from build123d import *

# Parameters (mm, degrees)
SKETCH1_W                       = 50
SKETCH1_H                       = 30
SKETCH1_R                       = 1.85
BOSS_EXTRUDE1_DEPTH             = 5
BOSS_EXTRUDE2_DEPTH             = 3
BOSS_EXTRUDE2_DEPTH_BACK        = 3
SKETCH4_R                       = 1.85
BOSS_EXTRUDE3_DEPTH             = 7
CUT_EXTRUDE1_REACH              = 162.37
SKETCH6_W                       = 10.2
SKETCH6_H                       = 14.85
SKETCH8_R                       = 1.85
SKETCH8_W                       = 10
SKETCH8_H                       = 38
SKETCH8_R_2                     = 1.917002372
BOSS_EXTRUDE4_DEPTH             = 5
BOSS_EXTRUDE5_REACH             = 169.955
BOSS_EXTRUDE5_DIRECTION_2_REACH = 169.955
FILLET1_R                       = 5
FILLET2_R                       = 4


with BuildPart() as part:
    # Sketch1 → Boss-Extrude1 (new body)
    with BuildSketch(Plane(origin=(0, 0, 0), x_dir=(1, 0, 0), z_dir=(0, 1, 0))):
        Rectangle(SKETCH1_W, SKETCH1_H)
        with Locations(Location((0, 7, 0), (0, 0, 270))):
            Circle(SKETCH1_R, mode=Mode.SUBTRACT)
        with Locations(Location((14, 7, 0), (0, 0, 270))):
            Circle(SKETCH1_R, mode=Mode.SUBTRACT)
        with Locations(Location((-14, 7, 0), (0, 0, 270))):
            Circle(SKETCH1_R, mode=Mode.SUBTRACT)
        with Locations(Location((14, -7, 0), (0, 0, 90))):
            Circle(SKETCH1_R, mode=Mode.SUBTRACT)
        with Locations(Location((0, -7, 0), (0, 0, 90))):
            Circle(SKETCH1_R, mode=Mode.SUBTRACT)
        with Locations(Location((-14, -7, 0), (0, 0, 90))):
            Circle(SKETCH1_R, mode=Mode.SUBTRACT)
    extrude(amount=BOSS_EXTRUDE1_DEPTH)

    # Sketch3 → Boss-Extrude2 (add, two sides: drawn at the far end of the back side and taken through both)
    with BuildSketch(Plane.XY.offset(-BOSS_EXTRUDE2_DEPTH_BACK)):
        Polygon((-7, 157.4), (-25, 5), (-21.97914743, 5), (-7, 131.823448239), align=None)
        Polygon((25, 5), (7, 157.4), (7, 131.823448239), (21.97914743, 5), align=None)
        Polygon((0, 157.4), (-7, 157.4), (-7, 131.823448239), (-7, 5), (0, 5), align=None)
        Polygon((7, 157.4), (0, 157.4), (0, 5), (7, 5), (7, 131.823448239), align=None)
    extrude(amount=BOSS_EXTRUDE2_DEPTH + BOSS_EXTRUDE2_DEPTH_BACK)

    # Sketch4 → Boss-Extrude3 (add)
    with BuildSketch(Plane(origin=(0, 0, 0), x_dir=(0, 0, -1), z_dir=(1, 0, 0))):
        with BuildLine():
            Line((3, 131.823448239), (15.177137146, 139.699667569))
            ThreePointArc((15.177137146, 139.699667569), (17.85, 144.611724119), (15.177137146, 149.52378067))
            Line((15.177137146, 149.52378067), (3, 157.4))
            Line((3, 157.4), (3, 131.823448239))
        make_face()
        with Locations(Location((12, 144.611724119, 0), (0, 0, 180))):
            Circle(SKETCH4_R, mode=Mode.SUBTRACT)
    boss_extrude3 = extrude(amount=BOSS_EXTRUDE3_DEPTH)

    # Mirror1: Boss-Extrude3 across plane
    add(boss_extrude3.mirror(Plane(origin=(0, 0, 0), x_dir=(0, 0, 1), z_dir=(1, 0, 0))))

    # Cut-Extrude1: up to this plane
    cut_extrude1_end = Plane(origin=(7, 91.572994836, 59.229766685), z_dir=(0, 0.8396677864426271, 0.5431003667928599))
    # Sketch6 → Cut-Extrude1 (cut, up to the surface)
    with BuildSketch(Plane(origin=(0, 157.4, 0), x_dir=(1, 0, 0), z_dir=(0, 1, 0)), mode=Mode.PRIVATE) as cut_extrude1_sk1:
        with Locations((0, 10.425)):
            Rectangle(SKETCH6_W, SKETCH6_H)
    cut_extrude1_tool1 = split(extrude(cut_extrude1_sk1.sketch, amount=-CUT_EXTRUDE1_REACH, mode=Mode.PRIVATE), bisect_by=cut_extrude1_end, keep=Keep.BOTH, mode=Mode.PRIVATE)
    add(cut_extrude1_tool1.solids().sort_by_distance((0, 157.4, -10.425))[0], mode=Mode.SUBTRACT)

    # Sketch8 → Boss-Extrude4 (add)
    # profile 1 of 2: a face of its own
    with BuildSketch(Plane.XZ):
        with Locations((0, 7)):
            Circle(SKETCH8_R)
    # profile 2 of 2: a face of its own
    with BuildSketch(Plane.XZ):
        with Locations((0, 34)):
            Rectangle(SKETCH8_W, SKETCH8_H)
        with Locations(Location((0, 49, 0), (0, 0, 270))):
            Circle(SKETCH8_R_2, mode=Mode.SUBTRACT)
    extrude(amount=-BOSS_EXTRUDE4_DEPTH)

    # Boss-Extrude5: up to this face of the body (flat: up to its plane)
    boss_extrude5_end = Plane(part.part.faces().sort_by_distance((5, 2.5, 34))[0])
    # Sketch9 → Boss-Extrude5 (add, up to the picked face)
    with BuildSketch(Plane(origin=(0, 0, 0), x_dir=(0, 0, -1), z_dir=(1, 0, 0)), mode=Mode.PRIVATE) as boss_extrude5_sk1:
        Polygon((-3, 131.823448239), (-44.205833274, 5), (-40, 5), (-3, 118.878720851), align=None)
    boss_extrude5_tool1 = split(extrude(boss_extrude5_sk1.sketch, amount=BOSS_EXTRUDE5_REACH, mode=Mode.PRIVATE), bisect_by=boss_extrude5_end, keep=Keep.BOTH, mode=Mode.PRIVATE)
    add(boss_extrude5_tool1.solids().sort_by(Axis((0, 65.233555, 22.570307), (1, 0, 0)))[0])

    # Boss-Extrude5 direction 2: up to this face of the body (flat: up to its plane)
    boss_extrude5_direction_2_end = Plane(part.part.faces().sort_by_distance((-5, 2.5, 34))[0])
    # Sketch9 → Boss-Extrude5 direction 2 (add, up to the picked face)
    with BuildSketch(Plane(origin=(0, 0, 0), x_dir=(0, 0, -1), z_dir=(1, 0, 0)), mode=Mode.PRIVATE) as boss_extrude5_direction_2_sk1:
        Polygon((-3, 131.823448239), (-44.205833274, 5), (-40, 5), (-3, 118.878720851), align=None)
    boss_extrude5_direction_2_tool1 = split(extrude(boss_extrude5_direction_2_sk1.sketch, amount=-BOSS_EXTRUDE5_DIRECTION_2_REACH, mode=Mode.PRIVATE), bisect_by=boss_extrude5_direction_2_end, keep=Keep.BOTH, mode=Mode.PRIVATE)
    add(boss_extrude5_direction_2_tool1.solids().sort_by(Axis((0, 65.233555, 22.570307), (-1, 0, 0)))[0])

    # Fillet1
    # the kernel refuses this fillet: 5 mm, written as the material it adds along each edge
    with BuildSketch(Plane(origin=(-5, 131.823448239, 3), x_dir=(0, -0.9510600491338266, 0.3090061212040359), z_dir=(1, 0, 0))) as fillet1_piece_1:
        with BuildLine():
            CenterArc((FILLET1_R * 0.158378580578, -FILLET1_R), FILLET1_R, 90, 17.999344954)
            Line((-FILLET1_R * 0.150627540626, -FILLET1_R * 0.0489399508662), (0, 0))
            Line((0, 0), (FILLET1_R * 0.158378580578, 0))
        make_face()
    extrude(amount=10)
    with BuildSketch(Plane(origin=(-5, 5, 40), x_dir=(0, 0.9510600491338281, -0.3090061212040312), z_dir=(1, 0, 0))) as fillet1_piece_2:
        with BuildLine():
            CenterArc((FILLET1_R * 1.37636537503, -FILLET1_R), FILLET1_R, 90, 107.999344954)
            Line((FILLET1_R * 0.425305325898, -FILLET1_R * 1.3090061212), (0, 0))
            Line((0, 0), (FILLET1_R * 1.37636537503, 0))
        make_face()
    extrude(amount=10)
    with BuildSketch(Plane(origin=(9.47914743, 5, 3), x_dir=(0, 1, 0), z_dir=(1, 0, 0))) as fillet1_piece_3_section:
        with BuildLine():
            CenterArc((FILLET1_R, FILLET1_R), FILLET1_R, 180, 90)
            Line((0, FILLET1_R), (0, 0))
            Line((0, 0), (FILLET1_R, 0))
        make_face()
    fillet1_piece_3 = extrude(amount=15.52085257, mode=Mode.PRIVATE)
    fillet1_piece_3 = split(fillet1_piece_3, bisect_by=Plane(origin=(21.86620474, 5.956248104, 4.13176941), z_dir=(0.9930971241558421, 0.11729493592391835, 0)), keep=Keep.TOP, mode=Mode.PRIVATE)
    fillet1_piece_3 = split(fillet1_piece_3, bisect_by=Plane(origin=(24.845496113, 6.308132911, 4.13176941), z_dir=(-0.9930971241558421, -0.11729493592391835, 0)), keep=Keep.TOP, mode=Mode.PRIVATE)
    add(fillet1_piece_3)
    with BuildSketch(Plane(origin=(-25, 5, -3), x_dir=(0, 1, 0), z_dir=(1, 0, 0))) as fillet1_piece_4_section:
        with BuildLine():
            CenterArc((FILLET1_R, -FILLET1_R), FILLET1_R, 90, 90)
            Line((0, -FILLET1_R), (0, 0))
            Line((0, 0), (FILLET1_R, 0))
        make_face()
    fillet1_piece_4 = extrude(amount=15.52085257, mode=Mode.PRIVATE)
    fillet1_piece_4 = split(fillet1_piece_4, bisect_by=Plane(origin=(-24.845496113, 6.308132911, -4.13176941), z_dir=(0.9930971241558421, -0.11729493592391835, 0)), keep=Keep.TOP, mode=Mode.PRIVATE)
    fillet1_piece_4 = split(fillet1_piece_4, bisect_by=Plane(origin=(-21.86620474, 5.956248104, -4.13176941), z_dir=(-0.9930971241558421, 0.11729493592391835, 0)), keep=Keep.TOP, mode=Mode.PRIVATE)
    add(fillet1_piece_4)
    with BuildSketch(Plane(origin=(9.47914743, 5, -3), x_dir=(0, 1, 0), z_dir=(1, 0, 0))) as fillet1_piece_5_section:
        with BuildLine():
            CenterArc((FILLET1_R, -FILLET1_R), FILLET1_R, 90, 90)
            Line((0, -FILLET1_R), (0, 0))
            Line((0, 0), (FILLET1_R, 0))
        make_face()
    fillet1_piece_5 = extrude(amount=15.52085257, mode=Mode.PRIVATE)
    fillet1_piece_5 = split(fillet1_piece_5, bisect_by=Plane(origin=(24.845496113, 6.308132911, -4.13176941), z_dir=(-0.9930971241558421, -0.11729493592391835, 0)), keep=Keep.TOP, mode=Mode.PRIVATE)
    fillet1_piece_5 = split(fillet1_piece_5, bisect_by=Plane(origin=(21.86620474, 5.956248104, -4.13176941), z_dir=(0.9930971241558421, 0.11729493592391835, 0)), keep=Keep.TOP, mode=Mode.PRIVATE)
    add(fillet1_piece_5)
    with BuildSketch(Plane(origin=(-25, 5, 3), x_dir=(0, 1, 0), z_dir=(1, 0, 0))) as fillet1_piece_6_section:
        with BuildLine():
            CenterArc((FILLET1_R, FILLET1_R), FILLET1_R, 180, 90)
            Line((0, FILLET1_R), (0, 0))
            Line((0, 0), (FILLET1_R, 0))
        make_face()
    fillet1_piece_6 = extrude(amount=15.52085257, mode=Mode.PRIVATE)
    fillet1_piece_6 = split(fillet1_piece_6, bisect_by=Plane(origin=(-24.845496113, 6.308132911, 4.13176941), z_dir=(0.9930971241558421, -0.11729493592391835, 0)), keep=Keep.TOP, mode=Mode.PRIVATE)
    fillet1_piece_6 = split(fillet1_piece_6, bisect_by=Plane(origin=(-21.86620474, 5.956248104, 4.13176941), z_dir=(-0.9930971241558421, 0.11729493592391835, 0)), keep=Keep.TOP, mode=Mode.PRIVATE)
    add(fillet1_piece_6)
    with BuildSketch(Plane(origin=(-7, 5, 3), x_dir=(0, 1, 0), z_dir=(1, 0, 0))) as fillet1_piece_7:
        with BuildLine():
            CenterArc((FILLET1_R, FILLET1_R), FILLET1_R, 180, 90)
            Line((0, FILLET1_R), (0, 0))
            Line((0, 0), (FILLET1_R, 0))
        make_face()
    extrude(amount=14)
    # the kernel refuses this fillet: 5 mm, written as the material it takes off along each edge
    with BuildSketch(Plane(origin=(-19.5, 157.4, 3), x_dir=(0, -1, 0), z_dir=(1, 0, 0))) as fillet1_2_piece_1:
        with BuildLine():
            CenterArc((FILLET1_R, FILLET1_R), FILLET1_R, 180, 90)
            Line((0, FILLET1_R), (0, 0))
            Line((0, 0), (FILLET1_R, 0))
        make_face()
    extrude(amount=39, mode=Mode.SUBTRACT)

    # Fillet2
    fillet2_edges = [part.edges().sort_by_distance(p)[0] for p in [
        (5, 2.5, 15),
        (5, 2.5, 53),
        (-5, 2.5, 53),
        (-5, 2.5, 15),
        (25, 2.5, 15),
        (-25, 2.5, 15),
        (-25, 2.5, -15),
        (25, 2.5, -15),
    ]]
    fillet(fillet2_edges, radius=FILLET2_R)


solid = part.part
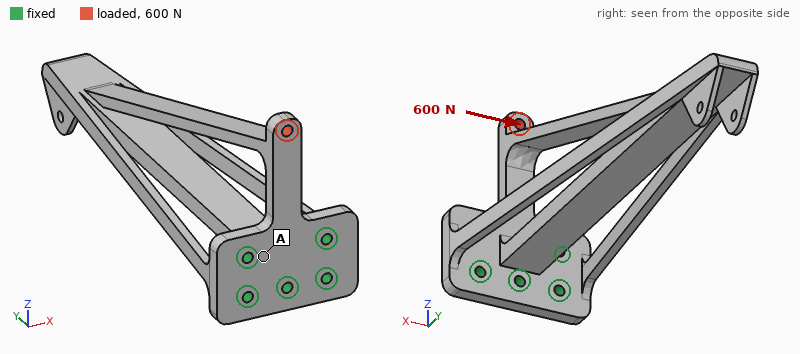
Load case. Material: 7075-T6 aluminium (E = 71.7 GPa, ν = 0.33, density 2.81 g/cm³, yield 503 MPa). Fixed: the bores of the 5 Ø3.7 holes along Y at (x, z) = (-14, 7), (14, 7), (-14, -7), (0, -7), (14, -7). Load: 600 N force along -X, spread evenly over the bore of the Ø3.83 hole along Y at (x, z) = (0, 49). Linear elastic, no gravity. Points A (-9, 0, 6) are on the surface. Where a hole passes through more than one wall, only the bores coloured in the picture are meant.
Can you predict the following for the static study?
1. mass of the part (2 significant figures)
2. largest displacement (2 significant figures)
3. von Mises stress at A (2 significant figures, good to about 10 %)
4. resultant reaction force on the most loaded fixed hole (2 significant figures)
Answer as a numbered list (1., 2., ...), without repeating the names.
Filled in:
1. 93 g
2. 0.35 mm
3. 19 MPa
4. 820 N
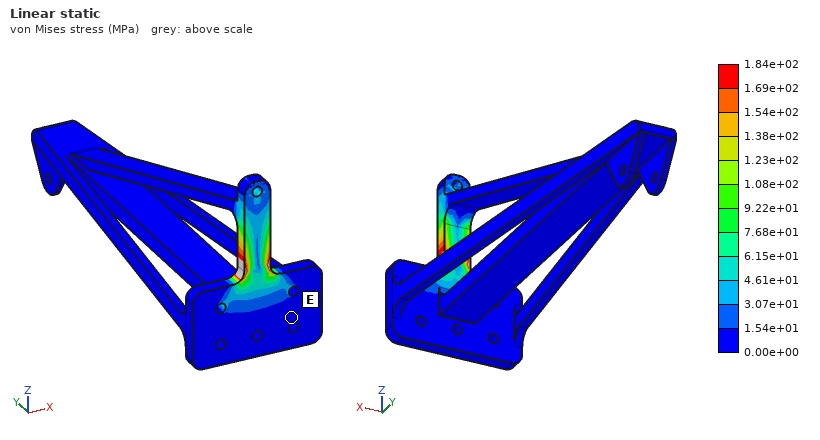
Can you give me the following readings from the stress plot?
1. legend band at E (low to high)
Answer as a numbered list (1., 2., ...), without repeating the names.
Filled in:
1. 0.00e+00 to 1.54e+01 MPa
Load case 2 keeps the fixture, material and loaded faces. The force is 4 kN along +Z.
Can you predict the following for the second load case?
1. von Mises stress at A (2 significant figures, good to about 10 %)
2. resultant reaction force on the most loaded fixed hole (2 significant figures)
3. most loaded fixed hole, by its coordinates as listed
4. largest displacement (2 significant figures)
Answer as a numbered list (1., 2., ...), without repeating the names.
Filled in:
1. 28 MPa
2. 1.3 kN
3. (0, -7)
4. 62 µm
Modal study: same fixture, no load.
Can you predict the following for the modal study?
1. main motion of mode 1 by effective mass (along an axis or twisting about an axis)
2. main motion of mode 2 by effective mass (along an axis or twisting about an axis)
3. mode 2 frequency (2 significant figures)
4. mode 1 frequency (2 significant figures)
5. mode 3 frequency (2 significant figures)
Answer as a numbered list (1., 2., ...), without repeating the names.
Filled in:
1. along Z
2. along X
3. 710 Hz
4. 310 Hz
5. 920 Hz
